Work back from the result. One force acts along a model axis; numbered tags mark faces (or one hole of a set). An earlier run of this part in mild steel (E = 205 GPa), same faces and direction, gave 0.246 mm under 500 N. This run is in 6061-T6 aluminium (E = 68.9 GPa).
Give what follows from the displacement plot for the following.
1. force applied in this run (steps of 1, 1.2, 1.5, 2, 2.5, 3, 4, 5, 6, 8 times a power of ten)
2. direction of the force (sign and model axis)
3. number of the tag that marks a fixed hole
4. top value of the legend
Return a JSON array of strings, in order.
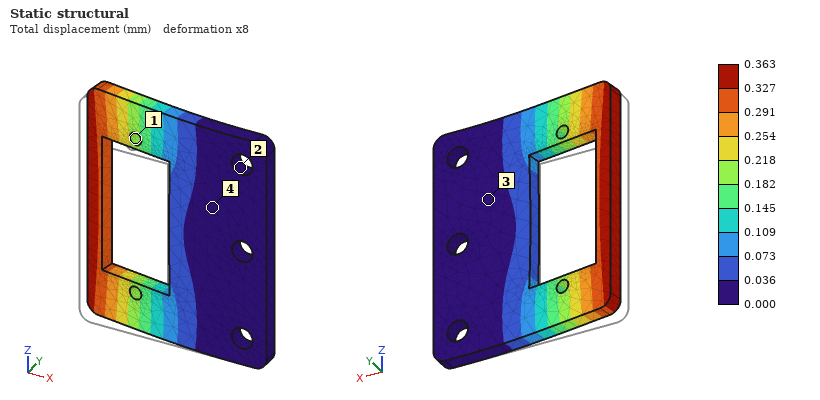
["250 N", "+Y", "2", "0.363 mm"]
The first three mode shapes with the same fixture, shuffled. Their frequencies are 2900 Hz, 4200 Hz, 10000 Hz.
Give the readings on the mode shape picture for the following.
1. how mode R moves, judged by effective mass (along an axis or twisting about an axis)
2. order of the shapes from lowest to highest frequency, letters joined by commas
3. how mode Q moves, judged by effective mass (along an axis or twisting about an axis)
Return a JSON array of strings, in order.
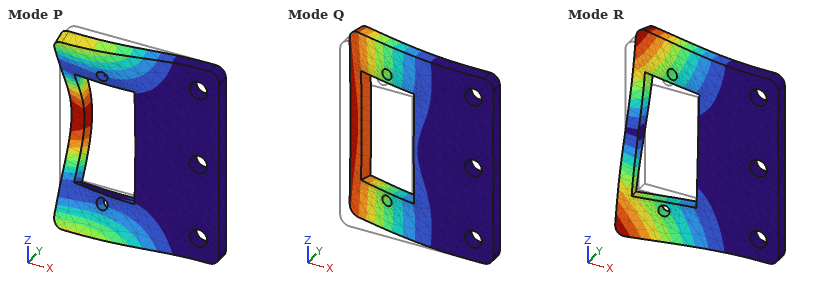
["twisting about X", "Q, R, P", "along Y"]
